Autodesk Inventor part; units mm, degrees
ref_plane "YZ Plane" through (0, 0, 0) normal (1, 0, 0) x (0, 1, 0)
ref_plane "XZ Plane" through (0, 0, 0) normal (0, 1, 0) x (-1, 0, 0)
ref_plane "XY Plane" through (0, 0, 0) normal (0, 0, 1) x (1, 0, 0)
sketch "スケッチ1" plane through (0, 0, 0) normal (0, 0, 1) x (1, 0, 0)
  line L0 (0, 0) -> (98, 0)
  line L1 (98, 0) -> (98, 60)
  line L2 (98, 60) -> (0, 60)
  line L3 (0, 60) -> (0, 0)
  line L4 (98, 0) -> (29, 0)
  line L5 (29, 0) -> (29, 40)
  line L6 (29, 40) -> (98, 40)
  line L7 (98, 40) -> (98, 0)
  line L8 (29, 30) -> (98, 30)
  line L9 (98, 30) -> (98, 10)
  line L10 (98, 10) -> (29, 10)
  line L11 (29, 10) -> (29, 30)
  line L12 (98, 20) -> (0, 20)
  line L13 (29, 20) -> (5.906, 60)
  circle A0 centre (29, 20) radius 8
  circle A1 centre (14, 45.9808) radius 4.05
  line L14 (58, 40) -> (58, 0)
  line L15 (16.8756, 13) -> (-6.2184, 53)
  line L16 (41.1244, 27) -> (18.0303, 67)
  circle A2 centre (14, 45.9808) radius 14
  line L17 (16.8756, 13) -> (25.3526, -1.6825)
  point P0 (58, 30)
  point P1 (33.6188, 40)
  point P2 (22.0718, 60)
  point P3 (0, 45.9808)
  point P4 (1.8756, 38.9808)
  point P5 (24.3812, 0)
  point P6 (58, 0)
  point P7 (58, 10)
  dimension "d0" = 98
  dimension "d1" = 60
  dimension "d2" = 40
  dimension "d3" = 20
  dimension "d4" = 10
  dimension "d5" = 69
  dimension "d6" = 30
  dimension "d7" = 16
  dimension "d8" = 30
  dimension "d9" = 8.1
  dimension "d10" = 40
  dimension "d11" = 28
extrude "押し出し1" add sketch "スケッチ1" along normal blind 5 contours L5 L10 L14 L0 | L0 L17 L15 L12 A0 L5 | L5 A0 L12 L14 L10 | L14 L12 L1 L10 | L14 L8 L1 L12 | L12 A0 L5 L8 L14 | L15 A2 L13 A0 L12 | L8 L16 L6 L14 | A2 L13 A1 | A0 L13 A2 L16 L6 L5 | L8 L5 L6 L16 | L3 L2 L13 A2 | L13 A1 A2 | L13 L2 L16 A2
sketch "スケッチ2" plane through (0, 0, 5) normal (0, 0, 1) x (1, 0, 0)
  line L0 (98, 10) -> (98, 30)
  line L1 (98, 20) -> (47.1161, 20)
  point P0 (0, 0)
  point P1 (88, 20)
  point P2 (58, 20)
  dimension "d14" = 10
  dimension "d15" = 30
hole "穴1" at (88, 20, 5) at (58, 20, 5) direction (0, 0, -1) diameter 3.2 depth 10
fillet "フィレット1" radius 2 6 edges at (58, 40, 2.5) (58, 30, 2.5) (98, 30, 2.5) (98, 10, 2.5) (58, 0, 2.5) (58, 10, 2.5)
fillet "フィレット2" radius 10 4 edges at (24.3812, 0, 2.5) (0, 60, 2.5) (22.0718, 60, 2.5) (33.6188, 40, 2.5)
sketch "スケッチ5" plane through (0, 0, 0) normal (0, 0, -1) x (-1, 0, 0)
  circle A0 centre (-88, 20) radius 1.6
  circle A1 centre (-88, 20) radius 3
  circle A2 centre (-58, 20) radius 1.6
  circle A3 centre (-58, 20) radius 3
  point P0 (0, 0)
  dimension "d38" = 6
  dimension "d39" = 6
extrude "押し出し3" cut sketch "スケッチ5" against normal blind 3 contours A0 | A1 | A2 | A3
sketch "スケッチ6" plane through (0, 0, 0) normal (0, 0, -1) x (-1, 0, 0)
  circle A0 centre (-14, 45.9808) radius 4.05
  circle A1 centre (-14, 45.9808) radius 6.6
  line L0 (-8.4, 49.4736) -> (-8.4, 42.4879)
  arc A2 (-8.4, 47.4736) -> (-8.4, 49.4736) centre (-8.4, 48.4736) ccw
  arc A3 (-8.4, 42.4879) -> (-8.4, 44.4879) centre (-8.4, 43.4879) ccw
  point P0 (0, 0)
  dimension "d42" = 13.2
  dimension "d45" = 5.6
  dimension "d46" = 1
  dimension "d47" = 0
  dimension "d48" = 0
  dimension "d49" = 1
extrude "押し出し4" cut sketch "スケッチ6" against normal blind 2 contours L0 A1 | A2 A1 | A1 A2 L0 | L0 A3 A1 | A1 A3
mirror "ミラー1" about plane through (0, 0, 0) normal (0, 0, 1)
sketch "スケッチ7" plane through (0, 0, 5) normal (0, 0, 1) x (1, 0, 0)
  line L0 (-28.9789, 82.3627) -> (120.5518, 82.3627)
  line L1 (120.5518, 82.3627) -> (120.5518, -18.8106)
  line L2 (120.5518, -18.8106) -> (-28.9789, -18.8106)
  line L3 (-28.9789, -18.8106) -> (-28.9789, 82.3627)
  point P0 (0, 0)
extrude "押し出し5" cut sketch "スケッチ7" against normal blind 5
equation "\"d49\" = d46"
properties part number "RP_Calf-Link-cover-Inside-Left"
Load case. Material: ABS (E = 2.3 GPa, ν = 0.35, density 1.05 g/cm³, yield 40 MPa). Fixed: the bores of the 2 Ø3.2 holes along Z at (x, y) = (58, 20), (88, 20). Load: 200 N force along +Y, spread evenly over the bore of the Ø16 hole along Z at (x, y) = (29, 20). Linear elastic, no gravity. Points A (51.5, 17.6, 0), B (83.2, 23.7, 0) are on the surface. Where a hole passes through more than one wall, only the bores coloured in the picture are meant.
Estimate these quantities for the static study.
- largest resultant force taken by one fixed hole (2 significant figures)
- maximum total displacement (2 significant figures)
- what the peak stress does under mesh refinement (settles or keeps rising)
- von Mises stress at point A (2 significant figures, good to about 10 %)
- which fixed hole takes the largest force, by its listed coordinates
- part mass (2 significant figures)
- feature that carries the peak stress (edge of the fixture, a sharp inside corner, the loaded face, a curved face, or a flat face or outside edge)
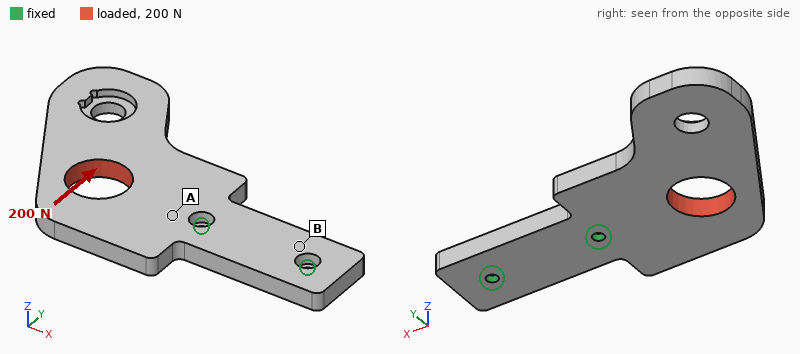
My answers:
370 N
1.3 mm
keeps rising
8.8 MPa
(58, 20)
15 g
edge of the fixture
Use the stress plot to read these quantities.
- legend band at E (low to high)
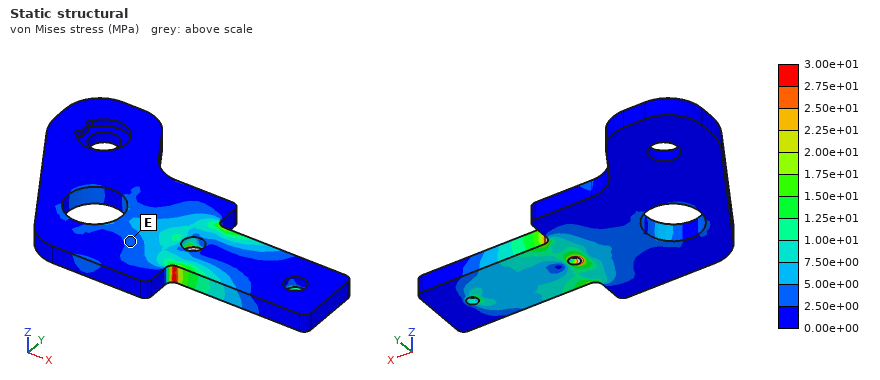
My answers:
2.50e+00 to 5.00e+00 MPa
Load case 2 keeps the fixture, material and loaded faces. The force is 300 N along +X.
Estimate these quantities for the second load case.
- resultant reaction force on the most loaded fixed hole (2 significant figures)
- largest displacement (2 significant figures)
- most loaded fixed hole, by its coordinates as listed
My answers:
210 N
0.26 mm
(58, 20)
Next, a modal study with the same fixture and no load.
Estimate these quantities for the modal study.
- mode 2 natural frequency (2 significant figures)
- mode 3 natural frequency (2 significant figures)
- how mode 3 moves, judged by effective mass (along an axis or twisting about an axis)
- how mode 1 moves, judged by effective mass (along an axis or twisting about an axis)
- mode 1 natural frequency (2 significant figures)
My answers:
590 Hz
800 Hz
along Y
along Z
240 Hz
